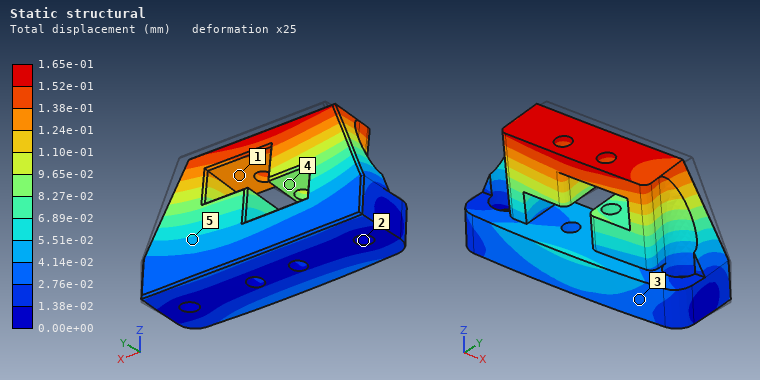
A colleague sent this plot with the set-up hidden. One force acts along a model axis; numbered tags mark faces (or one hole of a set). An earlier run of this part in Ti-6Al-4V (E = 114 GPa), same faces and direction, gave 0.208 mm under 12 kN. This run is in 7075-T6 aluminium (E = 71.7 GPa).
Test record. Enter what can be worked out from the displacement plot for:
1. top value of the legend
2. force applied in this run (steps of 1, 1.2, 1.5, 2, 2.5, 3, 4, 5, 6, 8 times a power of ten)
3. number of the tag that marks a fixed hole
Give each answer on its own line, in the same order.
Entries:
1.65e-01 mm
6 kN
2
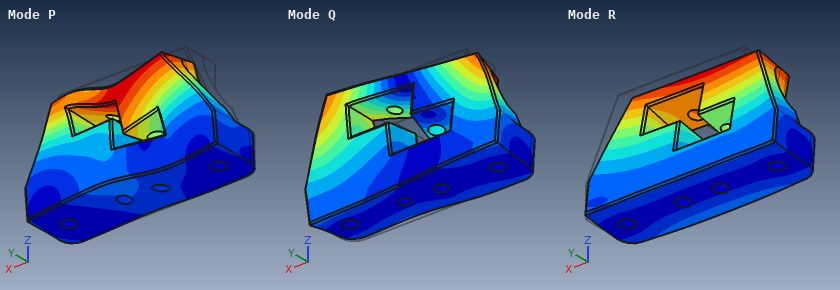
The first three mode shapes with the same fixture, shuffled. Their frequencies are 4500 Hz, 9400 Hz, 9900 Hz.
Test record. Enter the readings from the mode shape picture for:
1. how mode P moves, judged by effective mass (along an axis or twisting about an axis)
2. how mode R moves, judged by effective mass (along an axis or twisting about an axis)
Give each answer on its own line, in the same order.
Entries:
along X
along Y
